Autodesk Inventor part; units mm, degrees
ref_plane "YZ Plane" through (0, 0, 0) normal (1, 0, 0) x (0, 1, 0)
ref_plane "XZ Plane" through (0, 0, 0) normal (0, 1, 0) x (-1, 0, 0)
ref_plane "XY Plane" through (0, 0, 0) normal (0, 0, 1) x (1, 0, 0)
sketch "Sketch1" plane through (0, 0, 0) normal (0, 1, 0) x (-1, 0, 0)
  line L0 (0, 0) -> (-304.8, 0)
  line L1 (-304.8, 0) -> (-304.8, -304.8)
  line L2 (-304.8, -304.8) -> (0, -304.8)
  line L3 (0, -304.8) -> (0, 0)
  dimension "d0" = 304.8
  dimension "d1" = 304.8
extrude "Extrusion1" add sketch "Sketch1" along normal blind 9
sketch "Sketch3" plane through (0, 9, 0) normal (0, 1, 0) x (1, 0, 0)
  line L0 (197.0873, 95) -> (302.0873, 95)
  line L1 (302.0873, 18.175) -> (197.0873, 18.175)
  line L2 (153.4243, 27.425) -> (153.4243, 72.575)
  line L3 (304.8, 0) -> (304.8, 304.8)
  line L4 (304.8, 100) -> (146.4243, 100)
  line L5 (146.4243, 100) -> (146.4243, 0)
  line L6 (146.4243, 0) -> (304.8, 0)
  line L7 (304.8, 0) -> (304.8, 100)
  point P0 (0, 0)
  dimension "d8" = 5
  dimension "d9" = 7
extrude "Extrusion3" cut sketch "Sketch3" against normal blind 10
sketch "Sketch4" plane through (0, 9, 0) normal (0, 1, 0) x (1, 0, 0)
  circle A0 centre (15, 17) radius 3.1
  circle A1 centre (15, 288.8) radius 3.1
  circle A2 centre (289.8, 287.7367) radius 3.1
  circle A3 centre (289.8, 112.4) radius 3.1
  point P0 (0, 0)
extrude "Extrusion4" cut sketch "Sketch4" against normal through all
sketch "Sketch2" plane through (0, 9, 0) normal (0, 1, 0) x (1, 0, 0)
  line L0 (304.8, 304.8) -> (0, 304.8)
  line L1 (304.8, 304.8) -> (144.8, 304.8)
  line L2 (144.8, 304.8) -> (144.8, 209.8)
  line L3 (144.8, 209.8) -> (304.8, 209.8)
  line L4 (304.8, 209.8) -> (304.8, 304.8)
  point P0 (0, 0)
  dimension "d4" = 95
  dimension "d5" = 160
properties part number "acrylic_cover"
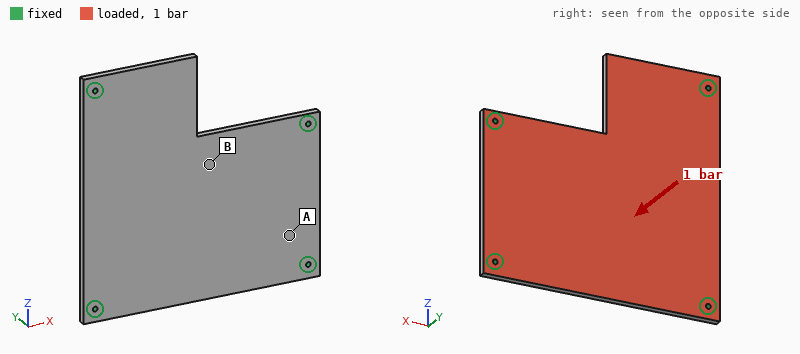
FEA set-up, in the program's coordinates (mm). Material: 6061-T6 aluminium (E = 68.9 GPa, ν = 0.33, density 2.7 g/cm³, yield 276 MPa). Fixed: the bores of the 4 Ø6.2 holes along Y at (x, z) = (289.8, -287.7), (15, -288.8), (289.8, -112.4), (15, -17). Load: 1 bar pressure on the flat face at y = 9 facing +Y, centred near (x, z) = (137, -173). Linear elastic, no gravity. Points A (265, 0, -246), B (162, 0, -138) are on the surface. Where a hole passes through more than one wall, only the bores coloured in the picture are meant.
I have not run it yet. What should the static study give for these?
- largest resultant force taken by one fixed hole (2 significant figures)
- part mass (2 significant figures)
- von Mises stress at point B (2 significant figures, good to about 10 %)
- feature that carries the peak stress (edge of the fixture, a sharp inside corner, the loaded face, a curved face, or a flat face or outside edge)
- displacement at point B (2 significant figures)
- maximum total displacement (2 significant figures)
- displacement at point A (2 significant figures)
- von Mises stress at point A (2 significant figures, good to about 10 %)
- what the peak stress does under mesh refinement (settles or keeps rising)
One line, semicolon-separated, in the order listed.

2.2 kN; 1.9 kg; 37 MPa; edge of the fixture; 0.92 mm; 1.0 mm; 0.21 mm; 15 MPa; keeps rising
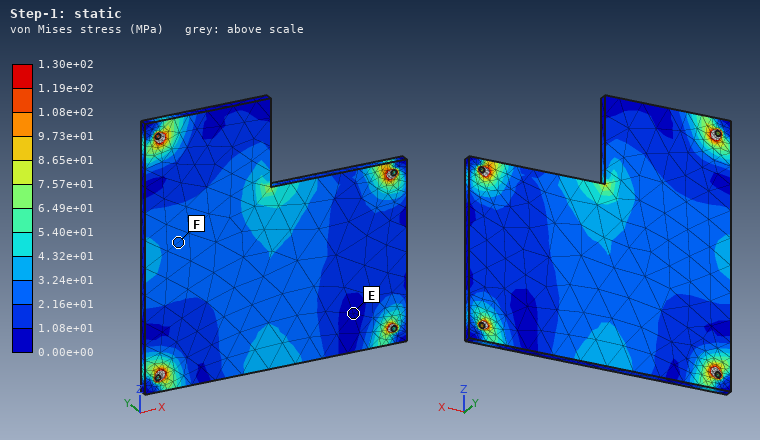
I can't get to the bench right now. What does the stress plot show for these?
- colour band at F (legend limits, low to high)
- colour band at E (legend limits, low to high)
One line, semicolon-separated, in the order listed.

2.16e+01 to 3.24e+01 MPa; 0.00e+00 to 1.08e+01 MPa
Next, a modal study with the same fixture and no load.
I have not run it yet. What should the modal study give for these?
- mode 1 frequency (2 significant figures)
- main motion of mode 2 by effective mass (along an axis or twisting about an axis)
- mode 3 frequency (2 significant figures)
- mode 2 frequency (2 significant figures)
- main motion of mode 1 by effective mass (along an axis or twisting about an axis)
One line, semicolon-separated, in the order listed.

390 Hz; twisting about X; 670 Hz; 620 Hz; along Y
